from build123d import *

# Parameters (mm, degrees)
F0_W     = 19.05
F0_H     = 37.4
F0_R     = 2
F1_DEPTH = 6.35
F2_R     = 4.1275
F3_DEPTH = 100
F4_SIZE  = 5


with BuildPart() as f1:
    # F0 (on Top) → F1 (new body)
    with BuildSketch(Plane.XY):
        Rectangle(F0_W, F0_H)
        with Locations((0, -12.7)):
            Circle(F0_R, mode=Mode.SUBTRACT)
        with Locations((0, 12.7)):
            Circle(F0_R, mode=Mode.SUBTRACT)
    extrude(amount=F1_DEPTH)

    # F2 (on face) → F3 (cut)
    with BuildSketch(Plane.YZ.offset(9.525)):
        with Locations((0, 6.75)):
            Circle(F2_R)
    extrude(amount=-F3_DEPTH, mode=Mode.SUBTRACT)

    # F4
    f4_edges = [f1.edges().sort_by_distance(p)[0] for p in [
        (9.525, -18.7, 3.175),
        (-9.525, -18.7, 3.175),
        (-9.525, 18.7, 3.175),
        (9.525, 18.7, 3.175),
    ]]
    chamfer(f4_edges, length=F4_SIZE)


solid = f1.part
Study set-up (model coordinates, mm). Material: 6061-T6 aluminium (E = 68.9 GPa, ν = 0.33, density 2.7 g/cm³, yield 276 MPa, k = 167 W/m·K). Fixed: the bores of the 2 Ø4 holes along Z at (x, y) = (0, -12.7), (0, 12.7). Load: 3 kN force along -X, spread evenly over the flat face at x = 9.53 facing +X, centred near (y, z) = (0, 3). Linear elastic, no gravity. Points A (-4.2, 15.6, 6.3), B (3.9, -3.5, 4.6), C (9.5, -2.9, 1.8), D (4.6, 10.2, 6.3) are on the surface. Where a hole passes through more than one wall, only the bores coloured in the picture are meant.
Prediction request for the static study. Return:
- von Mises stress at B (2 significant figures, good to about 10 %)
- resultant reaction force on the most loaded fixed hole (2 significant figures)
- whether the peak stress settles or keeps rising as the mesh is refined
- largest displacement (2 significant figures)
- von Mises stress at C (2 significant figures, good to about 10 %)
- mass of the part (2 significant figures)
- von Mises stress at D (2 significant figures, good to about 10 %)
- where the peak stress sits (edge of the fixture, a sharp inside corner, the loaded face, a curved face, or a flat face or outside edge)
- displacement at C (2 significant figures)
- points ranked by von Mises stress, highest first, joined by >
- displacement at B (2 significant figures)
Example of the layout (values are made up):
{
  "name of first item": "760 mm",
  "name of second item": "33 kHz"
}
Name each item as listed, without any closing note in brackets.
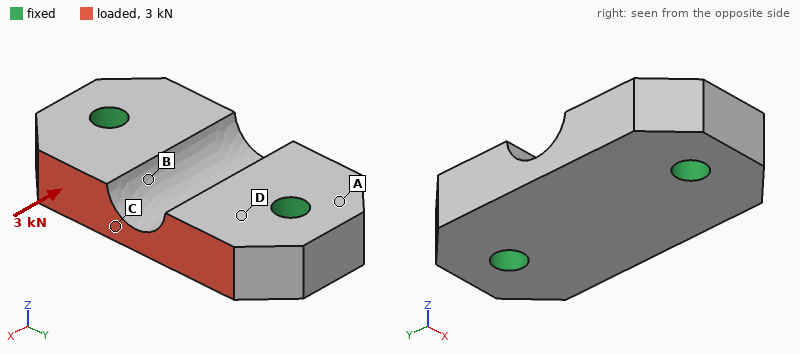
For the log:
{
  "von Mises stress at B": "15 MPa",
  "resultant reaction force on the most loaded fixed hole": "1.5 kN",
  "whether the peak stress settles or keeps rising as the mesh is refined": "keeps rising",
  "largest displacement": "9.1 µm",
  "von Mises stress at C": "33 MPa",
  "mass of the part": "9.7 g",
  "von Mises stress at D": "25 MPa",
  "where the peak stress sits": "edge of the fixture",
  "displacement at C": "7.5 µm",
  "points ranked by von Mises stress, highest first, joined by >": "C > D > B > A",
  "displacement at B": "5.3 µm"
}
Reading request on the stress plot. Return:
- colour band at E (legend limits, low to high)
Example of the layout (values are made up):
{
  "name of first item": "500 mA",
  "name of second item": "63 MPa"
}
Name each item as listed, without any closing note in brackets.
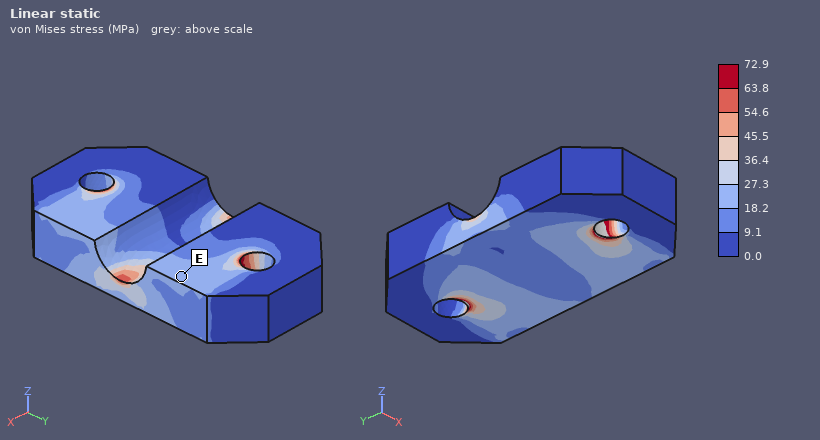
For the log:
{
  "colour band at E": "18.2 to 27.3 MPa"
}
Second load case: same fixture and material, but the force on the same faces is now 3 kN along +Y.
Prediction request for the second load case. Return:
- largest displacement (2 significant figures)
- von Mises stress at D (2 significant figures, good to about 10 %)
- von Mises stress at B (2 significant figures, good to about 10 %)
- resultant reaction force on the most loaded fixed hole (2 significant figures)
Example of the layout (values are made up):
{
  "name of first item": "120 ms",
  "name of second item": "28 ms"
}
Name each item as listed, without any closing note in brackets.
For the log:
{
  "largest displacement": "11 µm",
  "von Mises stress at D": "25 MPa",
  "von Mises stress at B": "33 MPa",
  "resultant reaction force on the most loaded fixed hole": "1.7 kN"
}
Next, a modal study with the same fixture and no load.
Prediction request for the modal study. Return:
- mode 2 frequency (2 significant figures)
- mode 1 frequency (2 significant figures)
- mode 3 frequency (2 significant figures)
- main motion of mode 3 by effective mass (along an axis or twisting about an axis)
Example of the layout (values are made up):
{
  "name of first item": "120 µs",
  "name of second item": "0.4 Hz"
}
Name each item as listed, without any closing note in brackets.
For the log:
{
  "mode 2 frequency": "35 kHz",
  "mode 1 frequency": "34 kHz",
  "mode 3 frequency": "46 kHz",
  "main motion of mode 3 by effective mass": "along X"
}
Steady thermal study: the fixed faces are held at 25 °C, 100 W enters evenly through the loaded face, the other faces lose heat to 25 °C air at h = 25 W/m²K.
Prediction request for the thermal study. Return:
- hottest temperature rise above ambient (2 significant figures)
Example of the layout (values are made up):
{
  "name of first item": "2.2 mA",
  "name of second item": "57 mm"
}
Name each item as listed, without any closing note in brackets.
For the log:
{
  "hottest temperature rise above ambient": "42 K"
}
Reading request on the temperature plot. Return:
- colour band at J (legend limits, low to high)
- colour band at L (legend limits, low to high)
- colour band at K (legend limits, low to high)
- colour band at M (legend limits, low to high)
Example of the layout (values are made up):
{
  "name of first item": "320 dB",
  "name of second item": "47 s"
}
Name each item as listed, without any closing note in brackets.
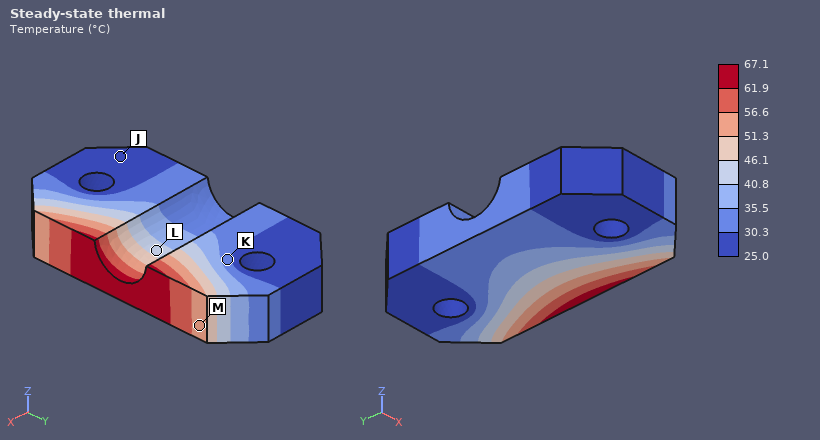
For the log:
{
  "colour band at J": "25.0 to 30.3 °C",
  "colour band at L": "40.8 to 46.1 °C",
  "colour band at K": "30.3 to 35.5 °C",
  "colour band at M": "51.3 to 56.6 °C"
}
